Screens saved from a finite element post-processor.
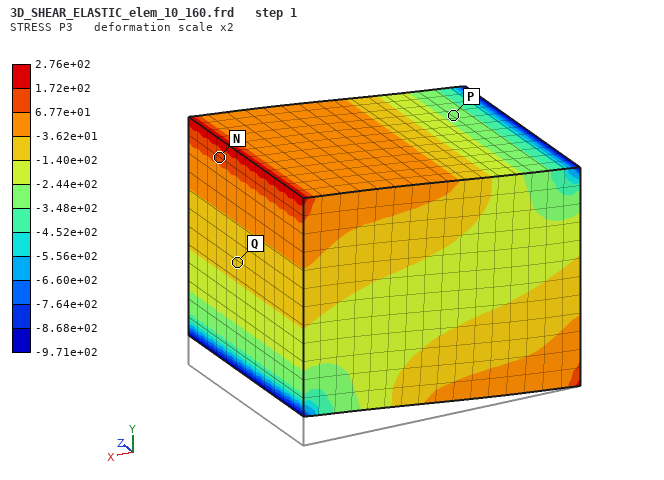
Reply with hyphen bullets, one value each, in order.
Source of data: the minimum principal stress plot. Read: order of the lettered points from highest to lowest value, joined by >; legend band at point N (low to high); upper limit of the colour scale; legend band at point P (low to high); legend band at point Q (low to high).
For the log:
- N > Q > P
- 6.77e+01 to 1.72e+02
- 2.76e+02
- -3.48e+02 to -2.44e+02
- -1.40e+02 to -3.62e+01
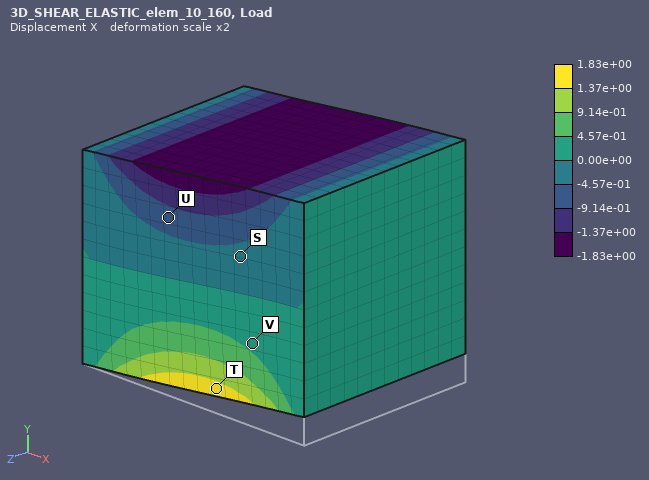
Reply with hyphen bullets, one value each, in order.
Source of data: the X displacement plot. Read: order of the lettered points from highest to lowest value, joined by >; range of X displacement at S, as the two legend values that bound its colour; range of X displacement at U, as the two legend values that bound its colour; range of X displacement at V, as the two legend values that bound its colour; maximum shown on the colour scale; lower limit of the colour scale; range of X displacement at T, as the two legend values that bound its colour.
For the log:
- T > V > S > U
- -4.57e-01 to 0.00e+00
- -9.14e-01 to -4.57e-01
- 0.00e+00 to 4.57e-01
- 1.83e+00
- -1.83e+00
- 1.37e+00 to 1.83e+00
